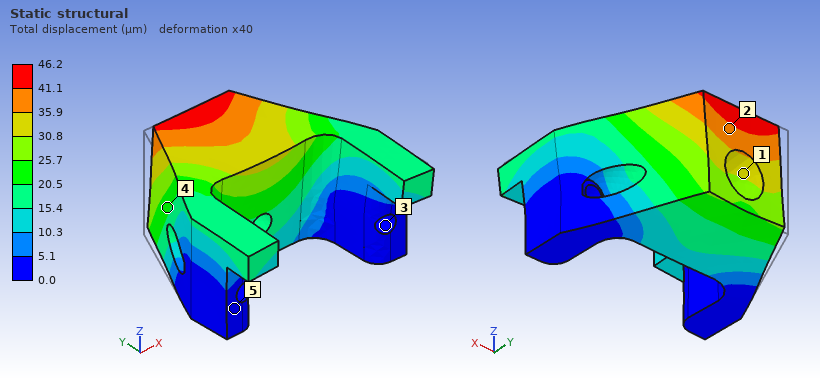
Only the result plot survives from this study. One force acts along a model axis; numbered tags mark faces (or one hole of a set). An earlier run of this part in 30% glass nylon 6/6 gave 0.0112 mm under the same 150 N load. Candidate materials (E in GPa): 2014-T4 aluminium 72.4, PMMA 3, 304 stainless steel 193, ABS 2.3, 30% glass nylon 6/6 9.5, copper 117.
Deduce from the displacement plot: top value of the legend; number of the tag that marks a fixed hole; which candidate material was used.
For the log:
46.2 µm
3
ABS
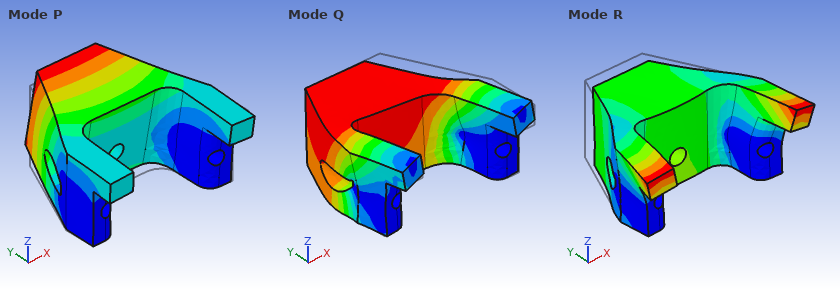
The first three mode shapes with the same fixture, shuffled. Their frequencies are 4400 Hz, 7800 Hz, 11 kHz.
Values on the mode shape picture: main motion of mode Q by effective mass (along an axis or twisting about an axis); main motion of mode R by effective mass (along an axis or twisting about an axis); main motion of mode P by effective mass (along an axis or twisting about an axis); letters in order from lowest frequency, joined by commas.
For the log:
along X
along Y
along Z
P, Q, R
